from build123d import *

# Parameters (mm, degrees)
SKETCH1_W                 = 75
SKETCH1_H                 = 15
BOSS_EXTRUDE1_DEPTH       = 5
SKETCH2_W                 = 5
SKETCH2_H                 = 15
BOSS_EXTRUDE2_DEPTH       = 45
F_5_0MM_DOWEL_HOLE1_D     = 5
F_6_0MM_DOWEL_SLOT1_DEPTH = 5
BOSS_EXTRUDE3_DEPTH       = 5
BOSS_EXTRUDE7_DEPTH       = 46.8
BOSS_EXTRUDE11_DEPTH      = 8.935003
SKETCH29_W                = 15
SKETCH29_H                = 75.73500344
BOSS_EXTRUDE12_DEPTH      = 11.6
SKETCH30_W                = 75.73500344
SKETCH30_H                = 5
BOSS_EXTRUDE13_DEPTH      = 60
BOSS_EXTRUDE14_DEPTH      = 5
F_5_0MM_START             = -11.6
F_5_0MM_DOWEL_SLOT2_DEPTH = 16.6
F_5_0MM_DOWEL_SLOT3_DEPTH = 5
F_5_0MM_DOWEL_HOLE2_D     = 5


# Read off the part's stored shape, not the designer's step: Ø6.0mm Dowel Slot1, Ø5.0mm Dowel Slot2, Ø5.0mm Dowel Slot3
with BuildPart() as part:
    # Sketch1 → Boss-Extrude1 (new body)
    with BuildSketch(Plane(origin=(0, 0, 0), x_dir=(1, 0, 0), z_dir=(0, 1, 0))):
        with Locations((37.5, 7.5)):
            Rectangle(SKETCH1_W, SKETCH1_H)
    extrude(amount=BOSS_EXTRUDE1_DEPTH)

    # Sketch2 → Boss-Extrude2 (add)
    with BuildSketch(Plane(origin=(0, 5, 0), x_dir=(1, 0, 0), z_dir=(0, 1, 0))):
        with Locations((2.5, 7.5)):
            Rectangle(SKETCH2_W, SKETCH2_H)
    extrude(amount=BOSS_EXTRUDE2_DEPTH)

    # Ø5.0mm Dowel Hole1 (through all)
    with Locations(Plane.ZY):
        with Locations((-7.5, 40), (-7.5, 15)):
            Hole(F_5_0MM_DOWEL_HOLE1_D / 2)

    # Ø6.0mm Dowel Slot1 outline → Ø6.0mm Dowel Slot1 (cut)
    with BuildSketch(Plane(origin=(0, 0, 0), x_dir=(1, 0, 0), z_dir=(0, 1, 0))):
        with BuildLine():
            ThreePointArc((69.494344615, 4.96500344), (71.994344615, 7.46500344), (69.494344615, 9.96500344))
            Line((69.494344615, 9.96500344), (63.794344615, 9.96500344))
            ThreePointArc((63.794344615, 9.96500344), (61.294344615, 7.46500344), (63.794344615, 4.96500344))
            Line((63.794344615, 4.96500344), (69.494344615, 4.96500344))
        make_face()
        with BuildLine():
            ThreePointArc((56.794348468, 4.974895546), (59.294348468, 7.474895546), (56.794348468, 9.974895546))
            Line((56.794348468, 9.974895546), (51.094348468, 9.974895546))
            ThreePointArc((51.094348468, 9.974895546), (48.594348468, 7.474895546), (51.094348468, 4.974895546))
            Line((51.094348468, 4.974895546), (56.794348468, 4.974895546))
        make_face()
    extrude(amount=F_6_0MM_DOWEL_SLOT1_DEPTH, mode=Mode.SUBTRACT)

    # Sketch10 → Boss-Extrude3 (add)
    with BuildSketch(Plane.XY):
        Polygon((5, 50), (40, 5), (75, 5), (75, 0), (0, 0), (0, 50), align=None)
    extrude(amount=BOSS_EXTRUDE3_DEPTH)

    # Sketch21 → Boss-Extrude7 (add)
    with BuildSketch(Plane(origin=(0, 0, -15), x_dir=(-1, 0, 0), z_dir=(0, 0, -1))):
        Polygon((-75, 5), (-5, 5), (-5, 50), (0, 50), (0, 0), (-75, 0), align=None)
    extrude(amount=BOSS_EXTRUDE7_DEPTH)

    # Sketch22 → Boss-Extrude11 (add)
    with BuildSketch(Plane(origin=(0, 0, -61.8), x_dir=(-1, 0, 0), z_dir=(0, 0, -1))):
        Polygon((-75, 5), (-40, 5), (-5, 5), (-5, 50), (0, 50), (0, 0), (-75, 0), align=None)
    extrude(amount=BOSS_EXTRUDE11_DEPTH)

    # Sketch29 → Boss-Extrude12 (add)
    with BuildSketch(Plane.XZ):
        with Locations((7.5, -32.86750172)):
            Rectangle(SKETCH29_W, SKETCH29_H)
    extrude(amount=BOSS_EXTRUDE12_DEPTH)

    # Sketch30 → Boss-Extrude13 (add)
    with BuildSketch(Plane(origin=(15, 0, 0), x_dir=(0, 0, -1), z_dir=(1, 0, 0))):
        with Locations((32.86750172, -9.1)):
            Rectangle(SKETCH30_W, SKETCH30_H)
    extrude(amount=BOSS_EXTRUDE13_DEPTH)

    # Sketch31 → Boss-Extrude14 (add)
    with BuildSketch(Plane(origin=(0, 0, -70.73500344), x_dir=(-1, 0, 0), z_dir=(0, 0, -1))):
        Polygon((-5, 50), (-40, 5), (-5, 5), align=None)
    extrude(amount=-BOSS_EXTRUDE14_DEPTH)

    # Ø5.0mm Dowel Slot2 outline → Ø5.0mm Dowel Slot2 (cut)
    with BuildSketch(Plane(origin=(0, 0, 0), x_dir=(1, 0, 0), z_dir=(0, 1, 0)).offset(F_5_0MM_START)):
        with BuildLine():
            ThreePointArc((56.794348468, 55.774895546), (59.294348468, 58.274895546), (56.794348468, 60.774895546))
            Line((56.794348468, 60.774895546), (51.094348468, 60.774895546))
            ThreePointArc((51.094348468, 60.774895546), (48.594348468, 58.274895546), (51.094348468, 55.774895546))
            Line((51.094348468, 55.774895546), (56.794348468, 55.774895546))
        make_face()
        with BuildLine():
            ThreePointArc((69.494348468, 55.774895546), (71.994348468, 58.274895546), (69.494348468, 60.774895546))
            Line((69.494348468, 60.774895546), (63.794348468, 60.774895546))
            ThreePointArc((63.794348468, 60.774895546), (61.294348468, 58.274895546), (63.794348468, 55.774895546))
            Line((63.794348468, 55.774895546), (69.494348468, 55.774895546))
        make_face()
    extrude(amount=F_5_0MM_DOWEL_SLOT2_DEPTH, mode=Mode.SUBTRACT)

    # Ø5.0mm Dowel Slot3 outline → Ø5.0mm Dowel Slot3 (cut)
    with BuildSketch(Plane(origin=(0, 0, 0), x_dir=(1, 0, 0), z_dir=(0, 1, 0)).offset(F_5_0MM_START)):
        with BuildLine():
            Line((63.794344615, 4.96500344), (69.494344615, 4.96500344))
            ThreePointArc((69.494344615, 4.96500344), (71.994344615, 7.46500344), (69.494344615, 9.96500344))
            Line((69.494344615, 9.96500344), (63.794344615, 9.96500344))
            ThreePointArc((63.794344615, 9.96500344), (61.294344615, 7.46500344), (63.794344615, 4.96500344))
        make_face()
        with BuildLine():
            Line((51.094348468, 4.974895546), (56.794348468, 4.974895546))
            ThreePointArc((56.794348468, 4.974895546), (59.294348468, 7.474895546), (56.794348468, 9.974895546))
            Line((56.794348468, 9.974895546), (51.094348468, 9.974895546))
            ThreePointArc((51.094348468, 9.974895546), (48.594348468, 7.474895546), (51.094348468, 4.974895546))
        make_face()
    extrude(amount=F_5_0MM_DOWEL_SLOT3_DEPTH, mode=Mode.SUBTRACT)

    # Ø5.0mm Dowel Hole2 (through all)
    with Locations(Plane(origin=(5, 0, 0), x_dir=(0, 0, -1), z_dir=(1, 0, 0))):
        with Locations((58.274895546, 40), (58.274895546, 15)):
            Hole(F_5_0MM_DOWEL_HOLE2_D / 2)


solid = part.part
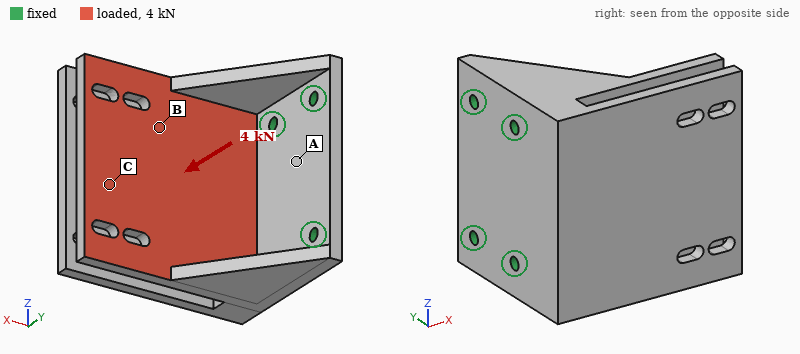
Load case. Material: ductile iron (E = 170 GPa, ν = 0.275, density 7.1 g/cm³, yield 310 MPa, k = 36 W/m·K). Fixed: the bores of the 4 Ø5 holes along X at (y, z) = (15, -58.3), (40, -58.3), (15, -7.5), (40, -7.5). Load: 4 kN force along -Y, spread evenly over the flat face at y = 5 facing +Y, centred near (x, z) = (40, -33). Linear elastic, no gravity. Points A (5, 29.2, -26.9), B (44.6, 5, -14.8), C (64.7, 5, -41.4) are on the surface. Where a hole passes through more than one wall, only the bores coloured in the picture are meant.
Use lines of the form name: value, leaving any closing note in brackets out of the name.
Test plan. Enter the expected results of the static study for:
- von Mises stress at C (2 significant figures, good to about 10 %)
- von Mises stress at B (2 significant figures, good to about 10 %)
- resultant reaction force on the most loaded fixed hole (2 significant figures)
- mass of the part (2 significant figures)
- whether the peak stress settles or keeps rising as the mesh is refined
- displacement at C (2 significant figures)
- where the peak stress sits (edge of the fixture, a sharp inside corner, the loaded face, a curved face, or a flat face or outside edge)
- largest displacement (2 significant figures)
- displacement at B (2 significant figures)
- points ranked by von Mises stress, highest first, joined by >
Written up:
von Mises stress at C: 54 MPa
von Mises stress at B: 97 MPa
resultant reaction force on the most loaded fixed hole: 2.9 kN
mass of the part: 620 g
whether the peak stress settles or keeps rising as the mesh is refined: keeps rising
displacement at C: 0.36 mm
where the peak stress sits: edge of the fixture
largest displacement: 0.47 mm
displacement at B: 0.16 mm
points ranked by von Mises stress, highest first, joined by >: B > C > A
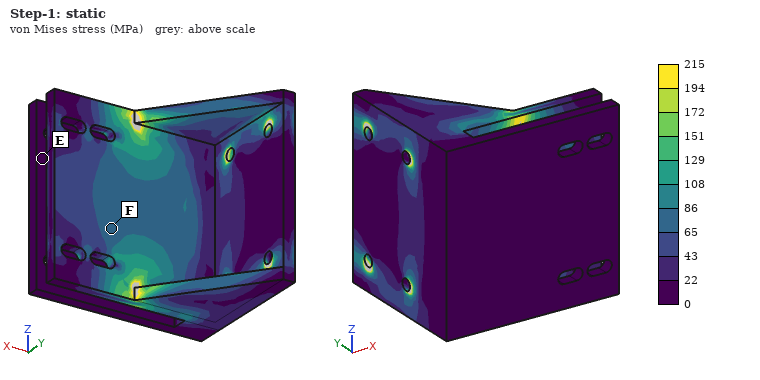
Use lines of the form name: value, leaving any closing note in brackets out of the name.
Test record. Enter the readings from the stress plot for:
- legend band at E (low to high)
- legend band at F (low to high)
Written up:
legend band at E: 0 to 22 MPa
legend band at F: 65 to 86 MPa
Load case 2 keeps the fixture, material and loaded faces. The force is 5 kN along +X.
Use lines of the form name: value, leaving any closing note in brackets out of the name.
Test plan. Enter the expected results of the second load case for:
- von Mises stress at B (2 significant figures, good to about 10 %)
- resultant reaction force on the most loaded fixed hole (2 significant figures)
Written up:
von Mises stress at B: 23 MPa
resultant reaction force on the most loaded fixed hole: 3.1 kN
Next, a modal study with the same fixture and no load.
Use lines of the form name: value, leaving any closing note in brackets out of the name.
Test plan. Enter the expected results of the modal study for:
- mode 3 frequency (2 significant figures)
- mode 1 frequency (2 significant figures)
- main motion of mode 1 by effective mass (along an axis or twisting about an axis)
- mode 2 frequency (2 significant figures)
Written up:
mode 3 frequency: 2000 Hz
mode 1 frequency: 930 Hz
main motion of mode 1 by effective mass: along Y
mode 2 frequency: 1500 Hz
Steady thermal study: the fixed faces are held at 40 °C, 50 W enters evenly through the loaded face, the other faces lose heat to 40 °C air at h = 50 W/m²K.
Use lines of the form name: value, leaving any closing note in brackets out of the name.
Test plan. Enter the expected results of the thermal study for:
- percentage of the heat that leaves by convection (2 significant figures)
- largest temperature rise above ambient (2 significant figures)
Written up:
percentage of the heat that leaves by convection: 62 %
largest temperature rise above ambient: 74 K
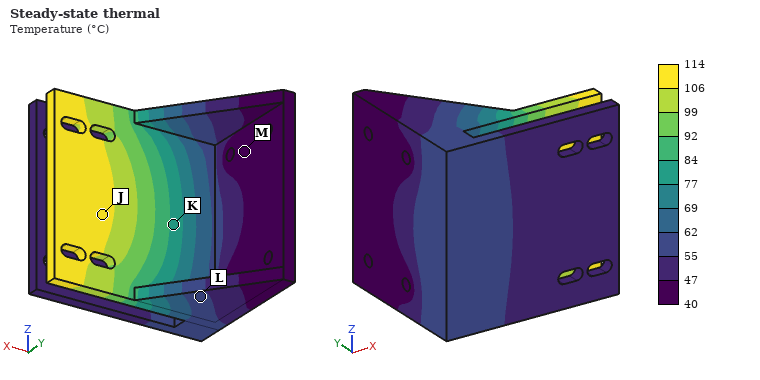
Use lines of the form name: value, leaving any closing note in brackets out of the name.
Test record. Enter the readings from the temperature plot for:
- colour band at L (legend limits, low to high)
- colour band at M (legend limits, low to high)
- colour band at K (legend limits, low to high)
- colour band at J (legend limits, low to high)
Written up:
colour band at L: 55 to 62 °C
colour band at M: 40 to 47 °C
colour band at K: 77 to 84 °C
colour band at J: 106 to 114 °C
